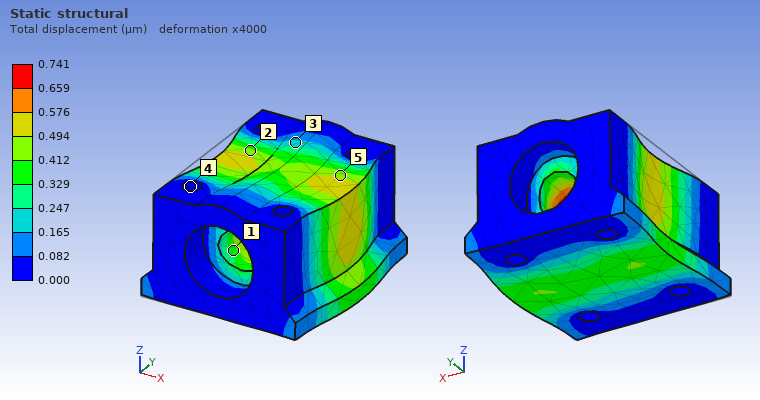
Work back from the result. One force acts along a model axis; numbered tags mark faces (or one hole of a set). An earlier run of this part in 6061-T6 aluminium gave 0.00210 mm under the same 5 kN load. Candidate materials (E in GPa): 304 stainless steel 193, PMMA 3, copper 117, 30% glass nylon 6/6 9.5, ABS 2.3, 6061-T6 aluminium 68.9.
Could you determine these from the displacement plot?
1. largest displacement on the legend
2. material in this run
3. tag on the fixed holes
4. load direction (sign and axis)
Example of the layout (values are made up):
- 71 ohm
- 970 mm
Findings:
- 0.741 µm
- 304 stainless steel
- 4
- +X
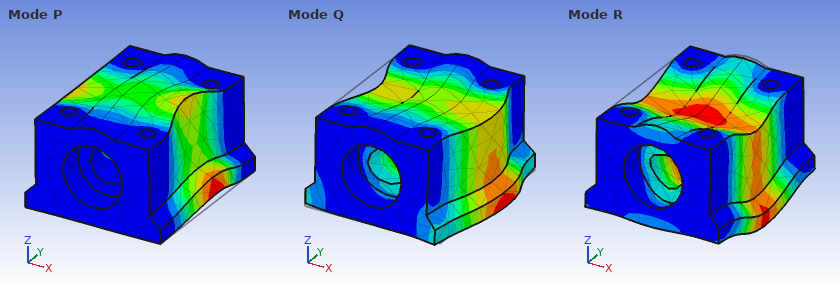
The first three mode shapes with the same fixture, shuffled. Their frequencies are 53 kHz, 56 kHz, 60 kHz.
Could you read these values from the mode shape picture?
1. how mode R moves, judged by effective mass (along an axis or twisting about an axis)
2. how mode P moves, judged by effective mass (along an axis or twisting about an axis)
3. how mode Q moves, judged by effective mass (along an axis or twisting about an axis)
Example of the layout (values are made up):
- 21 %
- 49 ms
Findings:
- along Z
- twisting about Y
- along X
